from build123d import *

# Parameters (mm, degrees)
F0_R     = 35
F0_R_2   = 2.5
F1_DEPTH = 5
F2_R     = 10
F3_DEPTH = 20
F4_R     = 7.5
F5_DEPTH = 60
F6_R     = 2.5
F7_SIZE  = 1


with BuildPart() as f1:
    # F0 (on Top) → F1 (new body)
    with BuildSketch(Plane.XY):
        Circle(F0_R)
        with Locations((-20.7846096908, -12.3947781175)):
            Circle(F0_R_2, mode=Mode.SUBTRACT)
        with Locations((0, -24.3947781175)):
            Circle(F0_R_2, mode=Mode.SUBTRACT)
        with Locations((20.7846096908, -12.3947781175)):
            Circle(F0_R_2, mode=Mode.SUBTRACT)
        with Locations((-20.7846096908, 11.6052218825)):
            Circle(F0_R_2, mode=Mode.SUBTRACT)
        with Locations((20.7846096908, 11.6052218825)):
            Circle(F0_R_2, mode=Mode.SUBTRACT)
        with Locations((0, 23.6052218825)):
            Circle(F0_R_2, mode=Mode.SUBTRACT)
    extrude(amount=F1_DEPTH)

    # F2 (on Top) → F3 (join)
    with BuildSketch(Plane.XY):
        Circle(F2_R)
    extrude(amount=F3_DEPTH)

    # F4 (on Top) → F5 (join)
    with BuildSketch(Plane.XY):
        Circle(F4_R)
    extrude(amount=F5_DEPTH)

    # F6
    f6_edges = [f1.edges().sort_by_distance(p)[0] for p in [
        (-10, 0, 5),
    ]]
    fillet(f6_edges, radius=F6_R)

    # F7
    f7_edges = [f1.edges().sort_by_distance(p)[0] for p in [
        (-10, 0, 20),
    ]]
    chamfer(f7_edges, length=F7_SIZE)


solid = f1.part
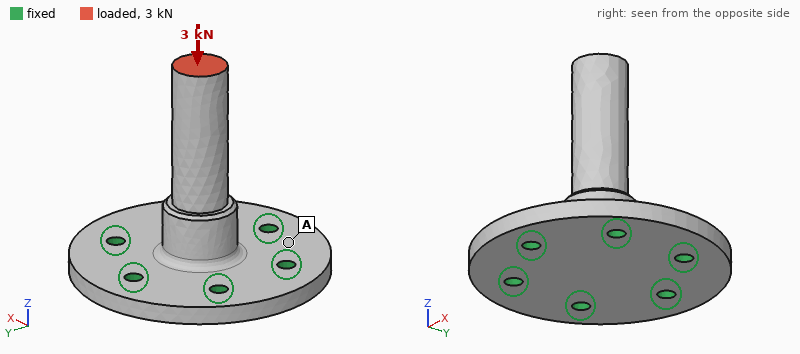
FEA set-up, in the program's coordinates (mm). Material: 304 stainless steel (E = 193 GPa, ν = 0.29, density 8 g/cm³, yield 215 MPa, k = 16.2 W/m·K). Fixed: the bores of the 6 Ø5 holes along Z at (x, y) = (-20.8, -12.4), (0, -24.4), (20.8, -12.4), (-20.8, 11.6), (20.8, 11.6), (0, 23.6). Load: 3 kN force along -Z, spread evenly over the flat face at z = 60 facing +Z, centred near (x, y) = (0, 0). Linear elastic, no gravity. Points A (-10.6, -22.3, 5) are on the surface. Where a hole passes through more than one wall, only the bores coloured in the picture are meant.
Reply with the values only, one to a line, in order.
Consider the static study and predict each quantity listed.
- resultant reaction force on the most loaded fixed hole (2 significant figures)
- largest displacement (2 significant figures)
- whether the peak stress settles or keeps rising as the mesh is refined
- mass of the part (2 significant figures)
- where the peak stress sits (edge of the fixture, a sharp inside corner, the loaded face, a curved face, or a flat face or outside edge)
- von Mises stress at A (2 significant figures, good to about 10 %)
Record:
560 N
10 µm
keeps rising
240 g
edge of the fixture
9.6 MPa
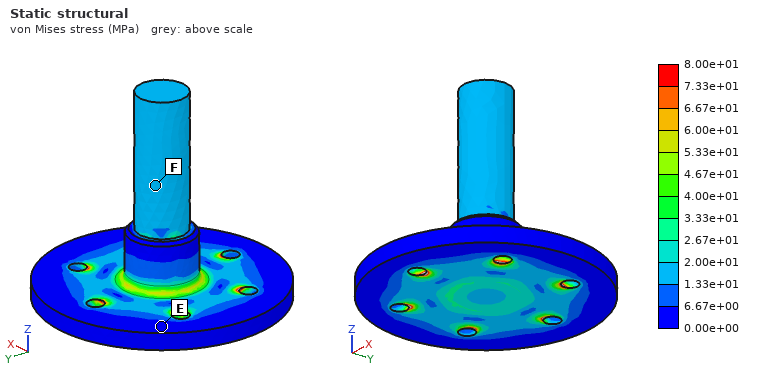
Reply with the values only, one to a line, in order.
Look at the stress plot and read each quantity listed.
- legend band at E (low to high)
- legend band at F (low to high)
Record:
0.00e+00 to 6.67e+00 MPa
1.33e+01 to 2.00e+01 MPa
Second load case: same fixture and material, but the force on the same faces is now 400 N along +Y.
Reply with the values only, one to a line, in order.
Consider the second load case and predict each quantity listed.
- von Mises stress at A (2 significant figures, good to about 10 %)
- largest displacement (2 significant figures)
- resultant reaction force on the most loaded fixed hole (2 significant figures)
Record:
5.3 MPa
46 µm
440 N
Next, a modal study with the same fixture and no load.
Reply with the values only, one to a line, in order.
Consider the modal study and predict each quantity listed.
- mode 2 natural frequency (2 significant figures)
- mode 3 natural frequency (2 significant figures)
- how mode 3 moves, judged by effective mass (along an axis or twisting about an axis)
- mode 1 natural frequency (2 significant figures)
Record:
3300 Hz
10 kHz
along Z
3300 Hz
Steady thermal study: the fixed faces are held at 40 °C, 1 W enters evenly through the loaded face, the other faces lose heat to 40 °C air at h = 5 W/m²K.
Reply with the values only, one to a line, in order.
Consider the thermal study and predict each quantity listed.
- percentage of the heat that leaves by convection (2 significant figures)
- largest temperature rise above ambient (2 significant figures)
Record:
14 %
18 K
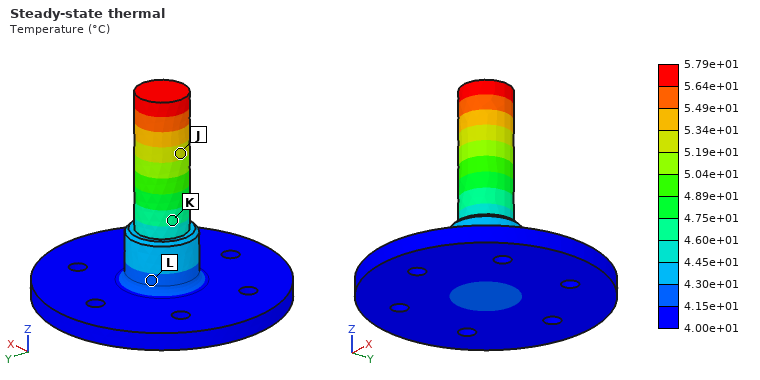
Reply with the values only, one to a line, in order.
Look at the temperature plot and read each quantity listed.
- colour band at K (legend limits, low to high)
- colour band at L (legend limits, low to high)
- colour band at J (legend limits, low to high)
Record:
4.60e+01 to 4.75e+01 °C
4.15e+01 to 4.30e+01 °C
5.19e+01 to 5.34e+01 °C
